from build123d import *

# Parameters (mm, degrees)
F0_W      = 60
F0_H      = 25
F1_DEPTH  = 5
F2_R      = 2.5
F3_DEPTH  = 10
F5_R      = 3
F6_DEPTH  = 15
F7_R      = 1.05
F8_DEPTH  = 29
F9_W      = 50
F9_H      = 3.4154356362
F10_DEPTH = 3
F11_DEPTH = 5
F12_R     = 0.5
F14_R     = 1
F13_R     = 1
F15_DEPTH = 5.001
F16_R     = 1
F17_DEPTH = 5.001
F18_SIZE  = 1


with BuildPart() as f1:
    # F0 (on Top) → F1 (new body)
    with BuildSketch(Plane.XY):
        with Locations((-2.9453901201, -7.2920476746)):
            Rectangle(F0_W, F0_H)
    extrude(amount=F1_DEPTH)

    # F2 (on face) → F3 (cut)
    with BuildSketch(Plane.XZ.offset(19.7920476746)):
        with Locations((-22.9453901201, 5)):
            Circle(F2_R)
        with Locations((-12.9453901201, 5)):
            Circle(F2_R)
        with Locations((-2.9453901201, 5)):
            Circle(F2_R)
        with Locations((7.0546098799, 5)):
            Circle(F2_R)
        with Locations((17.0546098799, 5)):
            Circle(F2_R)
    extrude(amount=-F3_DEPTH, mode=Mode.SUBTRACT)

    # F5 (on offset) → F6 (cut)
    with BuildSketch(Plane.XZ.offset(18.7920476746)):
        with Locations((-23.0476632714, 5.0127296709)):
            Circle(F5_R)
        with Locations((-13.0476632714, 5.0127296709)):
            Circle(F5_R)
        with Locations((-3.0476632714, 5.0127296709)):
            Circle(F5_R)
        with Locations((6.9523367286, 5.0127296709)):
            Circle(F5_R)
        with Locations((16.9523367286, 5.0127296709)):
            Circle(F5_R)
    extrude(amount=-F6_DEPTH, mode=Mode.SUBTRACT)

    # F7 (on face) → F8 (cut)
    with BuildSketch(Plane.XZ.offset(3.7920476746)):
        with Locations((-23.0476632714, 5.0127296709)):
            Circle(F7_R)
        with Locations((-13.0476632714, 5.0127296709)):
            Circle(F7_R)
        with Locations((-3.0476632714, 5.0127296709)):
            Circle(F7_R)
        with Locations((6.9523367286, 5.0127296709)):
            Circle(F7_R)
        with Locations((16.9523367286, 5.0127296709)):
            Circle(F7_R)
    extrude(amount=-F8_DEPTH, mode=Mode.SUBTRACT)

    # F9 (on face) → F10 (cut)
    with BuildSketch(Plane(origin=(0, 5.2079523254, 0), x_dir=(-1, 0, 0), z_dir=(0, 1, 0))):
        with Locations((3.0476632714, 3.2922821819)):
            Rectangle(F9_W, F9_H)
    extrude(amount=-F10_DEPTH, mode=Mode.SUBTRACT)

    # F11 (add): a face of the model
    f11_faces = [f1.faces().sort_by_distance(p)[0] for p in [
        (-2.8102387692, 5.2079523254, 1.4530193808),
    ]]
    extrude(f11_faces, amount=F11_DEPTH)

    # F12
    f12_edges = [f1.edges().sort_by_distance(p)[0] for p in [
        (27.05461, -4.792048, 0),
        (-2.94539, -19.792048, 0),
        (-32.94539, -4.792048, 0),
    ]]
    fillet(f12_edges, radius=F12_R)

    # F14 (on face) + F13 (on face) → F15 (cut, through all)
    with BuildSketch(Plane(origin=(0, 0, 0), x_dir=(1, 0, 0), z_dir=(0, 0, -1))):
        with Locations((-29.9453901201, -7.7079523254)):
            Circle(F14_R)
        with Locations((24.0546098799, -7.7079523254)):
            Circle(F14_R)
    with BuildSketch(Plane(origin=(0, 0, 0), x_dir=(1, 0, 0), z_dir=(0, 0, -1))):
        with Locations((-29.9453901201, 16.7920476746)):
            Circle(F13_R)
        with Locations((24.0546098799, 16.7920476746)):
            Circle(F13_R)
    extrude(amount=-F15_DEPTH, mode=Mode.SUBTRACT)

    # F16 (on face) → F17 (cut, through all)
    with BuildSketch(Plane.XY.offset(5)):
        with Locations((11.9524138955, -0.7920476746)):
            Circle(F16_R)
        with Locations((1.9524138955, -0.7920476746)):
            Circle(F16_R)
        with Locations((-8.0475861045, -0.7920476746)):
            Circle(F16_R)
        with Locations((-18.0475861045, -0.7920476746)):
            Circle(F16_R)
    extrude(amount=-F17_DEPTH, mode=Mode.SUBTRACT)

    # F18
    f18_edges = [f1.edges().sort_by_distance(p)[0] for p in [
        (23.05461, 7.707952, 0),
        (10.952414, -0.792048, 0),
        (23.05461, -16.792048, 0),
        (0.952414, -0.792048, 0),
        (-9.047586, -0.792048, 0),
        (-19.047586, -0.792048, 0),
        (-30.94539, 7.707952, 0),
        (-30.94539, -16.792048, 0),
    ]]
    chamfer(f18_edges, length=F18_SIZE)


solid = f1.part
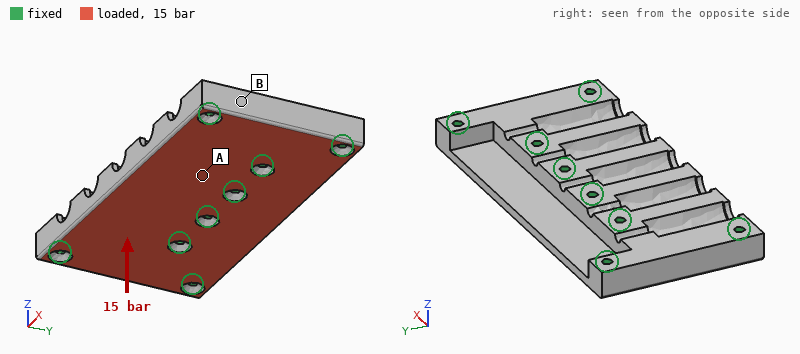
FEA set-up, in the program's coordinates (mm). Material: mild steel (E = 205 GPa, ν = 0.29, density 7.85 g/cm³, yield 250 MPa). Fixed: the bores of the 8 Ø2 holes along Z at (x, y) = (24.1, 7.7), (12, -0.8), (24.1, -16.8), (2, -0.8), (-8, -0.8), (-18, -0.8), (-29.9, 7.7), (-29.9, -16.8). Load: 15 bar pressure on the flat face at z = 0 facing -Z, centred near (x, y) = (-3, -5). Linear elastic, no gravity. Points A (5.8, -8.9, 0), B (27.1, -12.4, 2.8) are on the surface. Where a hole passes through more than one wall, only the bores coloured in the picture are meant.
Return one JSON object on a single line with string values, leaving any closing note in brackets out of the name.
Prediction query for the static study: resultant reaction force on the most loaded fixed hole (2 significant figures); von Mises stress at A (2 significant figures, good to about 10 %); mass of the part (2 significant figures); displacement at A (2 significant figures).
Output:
{"resultant reaction force on the most loaded fixed hole": "430 N", "von Mises stress at A": "18 MPa", "mass of the part": "50 g", "displacement at A": "3.8 µm"}
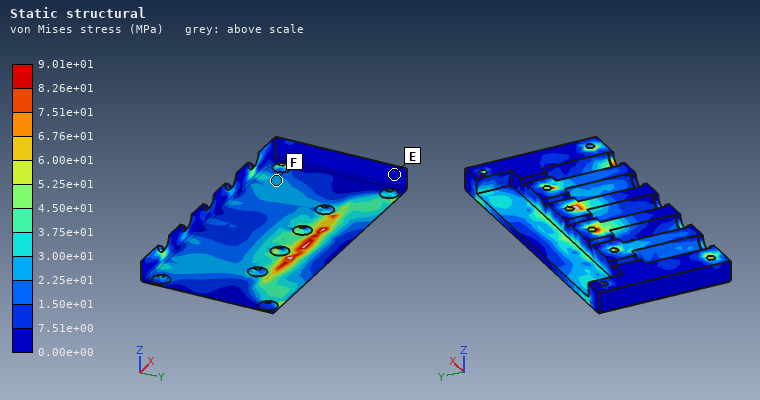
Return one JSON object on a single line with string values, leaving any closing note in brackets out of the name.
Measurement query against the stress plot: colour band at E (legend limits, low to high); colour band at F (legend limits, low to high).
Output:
{"colour band at E": "0.00e+00 to 7.51e+00 MPa", "colour band at F": "2.25e+01 to 3.00e+01 MPa"}
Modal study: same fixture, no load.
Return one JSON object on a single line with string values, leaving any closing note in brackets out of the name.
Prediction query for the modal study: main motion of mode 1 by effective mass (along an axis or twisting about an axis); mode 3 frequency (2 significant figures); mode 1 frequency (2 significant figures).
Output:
{"main motion of mode 1 by effective mass": "along Z", "mode 3 frequency": "21 kHz", "mode 1 frequency": "13 kHz"}
